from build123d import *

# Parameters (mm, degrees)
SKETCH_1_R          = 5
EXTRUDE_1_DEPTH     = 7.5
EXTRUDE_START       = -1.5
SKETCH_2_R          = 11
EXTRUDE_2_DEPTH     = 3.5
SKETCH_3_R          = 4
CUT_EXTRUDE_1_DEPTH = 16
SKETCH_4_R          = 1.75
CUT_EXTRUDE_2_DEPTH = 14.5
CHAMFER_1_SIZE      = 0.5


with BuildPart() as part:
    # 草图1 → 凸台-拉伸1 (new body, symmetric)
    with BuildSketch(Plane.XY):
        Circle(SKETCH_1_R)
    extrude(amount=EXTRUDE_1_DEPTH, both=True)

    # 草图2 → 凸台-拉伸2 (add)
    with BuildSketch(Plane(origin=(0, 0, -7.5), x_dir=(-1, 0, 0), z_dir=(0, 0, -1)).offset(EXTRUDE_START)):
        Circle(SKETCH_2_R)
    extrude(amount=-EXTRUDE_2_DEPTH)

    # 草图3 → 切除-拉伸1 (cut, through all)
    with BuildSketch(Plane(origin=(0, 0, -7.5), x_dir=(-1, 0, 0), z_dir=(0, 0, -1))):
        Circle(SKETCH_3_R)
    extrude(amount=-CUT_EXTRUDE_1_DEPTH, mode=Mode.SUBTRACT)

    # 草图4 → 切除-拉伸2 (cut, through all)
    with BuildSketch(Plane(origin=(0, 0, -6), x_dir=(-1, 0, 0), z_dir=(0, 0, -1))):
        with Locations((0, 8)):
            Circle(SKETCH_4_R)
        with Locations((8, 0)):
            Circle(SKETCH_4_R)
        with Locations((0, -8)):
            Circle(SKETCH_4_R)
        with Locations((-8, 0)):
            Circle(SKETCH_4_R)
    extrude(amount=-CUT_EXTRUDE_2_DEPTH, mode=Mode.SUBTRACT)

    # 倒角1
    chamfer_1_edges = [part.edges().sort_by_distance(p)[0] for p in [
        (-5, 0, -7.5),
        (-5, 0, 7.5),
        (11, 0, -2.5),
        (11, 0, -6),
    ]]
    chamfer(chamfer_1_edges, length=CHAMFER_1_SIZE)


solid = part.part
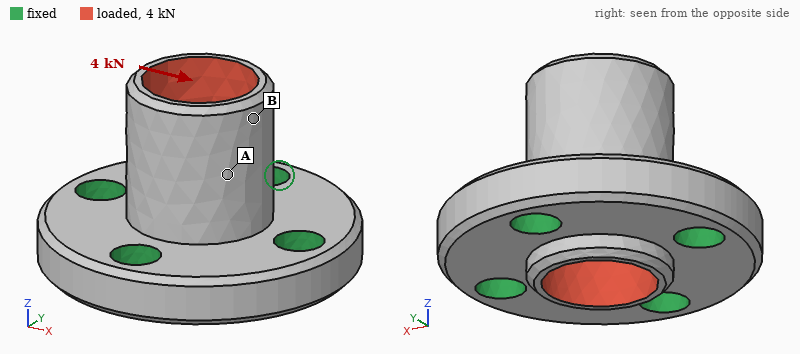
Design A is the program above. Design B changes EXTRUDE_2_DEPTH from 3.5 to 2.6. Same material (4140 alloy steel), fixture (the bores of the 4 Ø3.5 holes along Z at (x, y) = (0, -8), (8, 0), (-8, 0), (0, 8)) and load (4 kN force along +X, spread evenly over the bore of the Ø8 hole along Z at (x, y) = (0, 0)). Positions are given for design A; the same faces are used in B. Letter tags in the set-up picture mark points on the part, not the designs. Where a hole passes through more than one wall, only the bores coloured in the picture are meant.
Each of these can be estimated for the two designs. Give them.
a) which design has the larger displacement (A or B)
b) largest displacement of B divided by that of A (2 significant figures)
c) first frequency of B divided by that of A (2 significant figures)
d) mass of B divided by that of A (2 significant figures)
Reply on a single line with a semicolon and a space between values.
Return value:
B; 1.3; 0.86; 0.82
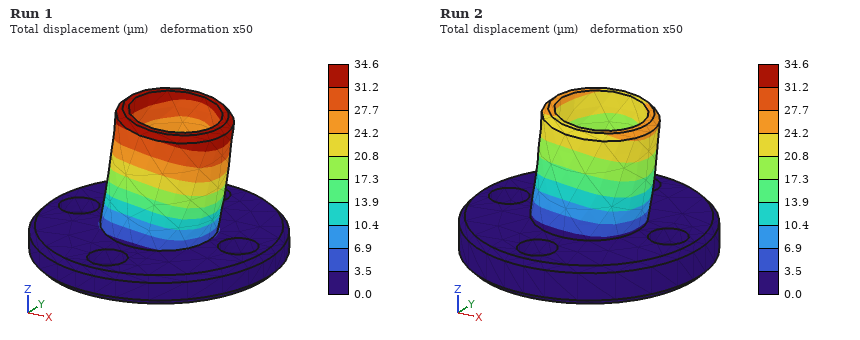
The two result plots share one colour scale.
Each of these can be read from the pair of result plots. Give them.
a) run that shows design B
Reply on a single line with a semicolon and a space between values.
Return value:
Run 1
